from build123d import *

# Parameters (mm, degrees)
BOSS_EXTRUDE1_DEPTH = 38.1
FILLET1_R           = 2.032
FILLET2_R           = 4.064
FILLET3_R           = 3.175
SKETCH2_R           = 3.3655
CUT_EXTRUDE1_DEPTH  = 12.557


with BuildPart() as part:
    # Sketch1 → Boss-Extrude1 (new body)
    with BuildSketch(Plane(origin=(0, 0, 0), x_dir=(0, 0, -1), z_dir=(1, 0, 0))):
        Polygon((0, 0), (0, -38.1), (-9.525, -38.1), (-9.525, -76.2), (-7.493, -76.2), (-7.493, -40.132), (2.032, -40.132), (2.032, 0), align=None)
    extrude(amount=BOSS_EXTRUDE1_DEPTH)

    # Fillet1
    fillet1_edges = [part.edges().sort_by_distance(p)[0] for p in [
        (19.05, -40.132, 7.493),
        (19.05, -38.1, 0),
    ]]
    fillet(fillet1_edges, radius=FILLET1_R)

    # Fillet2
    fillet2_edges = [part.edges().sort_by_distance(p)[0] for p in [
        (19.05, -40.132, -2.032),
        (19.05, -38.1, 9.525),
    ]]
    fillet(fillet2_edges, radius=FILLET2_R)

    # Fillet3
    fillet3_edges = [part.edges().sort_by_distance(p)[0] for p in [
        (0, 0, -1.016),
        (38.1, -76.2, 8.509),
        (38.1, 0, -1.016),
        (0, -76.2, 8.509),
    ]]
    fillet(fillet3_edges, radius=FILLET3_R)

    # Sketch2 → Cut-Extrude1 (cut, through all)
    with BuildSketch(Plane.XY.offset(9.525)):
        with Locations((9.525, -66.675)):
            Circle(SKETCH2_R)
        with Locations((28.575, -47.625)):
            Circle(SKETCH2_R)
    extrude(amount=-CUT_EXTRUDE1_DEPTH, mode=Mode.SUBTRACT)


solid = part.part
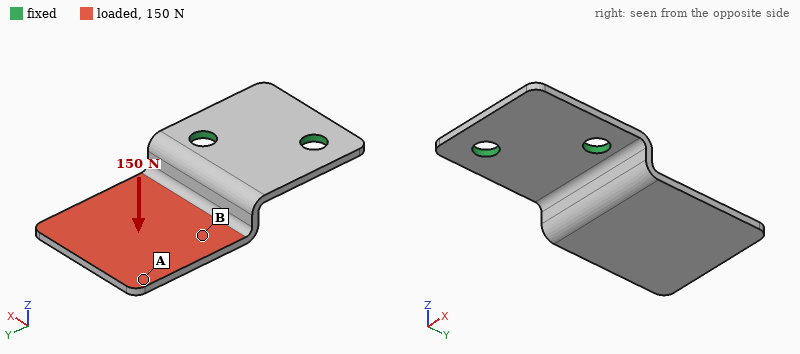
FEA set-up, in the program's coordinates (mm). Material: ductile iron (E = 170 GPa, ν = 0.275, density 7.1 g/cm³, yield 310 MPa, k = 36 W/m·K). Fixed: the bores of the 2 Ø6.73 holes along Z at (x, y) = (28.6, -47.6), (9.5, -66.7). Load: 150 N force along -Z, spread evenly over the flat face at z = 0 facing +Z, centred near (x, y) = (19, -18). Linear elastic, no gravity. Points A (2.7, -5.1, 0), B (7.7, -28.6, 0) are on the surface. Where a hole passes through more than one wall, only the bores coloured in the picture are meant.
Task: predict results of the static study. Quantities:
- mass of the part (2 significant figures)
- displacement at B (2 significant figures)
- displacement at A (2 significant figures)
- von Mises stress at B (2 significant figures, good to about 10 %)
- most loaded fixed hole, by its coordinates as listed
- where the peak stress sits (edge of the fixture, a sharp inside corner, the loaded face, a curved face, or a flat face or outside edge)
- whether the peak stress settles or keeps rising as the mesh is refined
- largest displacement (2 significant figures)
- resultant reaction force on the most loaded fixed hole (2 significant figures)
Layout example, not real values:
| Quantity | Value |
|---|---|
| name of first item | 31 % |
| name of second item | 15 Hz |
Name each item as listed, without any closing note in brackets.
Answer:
| Quantity | Value |
|---|---|
| mass of the part | 45 g |
| displacement at B | 0.24 mm |
| displacement at A | 0.69 mm |
| von Mises stress at B | 57 MPa |
| most loaded fixed hole, by its coordinates as listed | (28.6, -47.6) |
| where the peak stress sits | edge of the fixture |
| whether the peak stress settles or keeps rising as the mesh is refined | keeps rising |
| largest displacement | 0.80 mm |
| resultant reaction force on the most loaded fixed hole | 210 N |
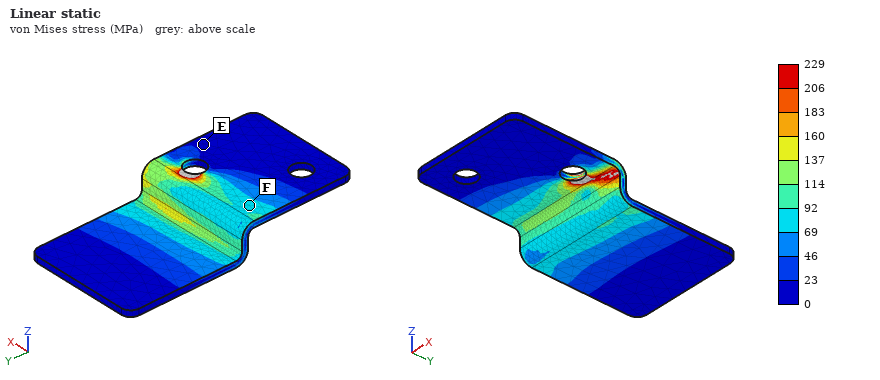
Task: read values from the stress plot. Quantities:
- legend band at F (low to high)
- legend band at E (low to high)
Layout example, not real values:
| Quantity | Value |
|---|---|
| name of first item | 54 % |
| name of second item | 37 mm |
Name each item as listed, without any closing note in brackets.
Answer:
| Quantity | Value |
|---|---|
| legend band at F | 69 to 92 MPa |
| legend band at E | 0 to 23 MPa |
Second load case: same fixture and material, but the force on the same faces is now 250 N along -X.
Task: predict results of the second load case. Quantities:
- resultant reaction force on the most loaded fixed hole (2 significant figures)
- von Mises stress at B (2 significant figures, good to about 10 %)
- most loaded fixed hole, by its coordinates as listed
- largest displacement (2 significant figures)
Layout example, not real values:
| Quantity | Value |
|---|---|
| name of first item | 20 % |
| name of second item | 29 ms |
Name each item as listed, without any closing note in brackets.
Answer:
| Quantity | Value |
|---|---|
| resultant reaction force on the most loaded fixed hole | 390 N |
| von Mises stress at B | 33 MPa |
| most loaded fixed hole, by its coordinates as listed | (28.6, -47.6) |
| largest displacement | 0.11 mm |
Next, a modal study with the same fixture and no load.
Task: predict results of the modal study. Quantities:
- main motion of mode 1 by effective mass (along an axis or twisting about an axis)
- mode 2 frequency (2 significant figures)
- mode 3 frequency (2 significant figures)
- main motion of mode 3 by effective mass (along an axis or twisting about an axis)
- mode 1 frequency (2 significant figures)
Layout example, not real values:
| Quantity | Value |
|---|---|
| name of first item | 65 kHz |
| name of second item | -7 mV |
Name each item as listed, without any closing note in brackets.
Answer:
| Quantity | Value |
|---|---|
| main motion of mode 1 by effective mass | along Z |
| mode 2 frequency | 1700 Hz |
| mode 3 frequency | 2400 Hz |
| main motion of mode 3 by effective mass | along X |
| mode 1 frequency | 610 Hz |
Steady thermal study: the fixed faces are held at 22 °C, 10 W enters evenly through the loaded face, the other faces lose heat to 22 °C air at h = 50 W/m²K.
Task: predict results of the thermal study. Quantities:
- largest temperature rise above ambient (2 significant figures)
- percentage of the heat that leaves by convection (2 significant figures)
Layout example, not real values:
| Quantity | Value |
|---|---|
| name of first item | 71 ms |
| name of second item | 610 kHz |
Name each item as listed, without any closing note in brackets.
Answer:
| Quantity | Value |
|---|---|
| largest temperature rise above ambient | 66 K |
| percentage of the heat that leaves by convection | 62 % |
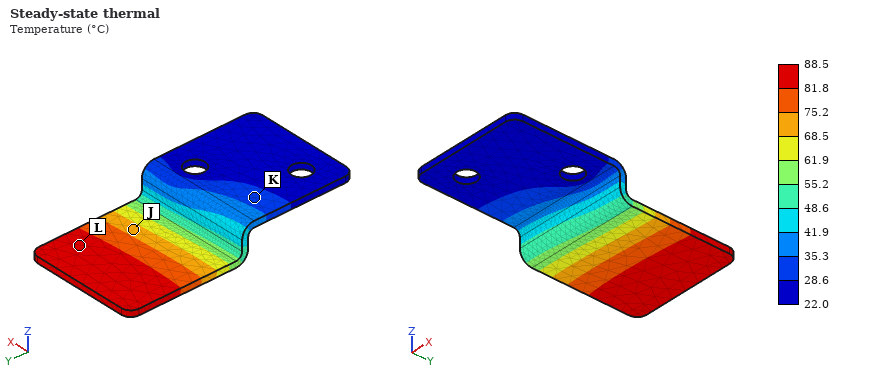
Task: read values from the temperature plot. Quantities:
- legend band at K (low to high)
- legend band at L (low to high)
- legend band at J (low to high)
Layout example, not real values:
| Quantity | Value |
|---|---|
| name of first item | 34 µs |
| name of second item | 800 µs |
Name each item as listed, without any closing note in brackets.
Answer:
| Quantity | Value |
|---|---|
| legend band at K | 28.6 to 35.3 °C |
| legend band at L | 81.8 to 88.5 °C |
| legend band at J | 68.5 to 75.2 °C |
